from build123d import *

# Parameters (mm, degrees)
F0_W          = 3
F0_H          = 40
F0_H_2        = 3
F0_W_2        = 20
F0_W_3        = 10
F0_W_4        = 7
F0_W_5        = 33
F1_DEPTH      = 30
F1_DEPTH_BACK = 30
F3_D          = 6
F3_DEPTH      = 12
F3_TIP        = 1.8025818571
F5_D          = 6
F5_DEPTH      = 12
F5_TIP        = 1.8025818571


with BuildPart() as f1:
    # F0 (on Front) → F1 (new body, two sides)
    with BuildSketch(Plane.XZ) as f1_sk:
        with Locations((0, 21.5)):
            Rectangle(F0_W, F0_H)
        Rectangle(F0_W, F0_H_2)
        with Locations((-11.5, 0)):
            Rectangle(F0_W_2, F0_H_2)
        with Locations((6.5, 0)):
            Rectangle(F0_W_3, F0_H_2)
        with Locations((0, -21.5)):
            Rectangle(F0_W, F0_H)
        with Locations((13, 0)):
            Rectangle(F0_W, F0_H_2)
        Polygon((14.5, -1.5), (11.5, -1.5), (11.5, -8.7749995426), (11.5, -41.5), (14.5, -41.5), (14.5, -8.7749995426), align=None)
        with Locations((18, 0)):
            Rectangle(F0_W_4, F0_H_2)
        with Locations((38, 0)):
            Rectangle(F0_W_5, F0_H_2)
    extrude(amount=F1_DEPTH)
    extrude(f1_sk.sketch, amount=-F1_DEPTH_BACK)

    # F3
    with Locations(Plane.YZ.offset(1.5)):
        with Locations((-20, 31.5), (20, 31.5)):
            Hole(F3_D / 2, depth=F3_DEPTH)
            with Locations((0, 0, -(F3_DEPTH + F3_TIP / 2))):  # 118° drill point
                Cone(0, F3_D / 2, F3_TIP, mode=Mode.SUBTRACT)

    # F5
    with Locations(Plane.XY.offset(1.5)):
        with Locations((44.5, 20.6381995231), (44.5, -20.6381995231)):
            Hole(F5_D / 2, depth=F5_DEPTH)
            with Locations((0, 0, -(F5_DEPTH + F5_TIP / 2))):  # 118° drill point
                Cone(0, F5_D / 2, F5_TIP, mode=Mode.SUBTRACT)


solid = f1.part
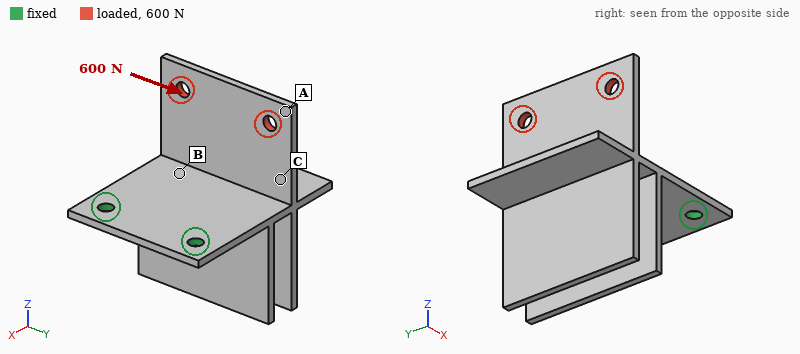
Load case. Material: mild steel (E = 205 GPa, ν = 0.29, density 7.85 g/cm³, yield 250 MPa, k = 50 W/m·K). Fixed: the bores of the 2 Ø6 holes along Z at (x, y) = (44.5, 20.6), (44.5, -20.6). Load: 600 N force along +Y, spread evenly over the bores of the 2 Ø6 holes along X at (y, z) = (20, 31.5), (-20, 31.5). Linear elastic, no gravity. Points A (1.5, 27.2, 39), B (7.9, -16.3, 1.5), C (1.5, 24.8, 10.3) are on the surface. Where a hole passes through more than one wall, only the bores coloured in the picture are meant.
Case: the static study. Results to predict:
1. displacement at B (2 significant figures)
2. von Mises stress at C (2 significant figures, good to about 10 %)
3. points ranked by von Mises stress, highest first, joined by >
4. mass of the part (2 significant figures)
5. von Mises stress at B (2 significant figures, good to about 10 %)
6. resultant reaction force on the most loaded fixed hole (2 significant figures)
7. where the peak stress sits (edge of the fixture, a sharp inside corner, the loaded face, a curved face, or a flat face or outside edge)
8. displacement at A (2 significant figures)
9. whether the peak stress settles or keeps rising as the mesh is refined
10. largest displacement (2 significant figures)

0.10 mm
34 MPa
B > C > A
270 g
80 MPa
790 N
edge of the fixture
0.36 mm
keeps rising
0.38 mm
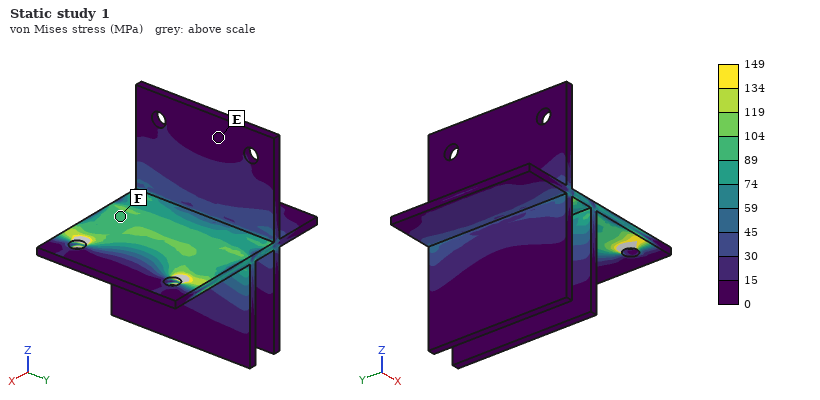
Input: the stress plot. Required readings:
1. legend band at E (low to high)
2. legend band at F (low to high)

0 to 15 MPa
89 to 104 MPa
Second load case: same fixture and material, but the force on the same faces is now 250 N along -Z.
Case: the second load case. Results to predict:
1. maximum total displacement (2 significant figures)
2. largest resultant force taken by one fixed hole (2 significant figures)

0.44 mm
130 N
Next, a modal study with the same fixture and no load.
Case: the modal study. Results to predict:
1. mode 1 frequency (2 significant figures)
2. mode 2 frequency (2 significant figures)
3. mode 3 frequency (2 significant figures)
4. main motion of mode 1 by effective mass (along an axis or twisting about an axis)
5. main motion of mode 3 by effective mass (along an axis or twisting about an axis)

280 Hz
670 Hz
990 Hz
along Z
along Z
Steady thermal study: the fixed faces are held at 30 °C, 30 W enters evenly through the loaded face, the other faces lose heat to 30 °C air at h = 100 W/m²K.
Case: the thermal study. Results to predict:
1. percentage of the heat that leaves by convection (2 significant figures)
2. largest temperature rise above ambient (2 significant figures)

97 %
78 K
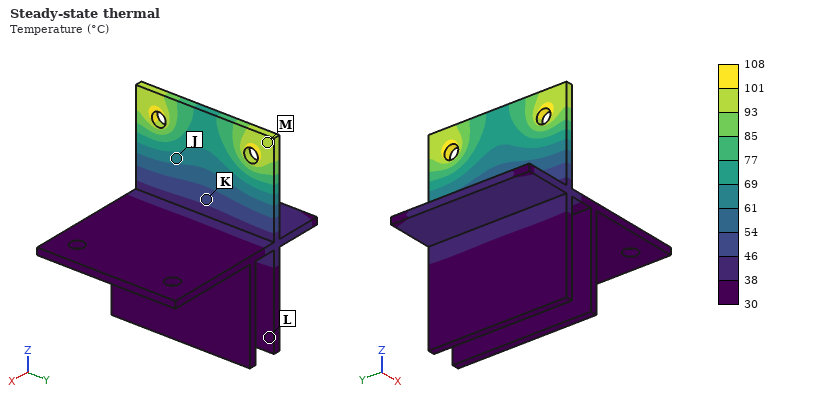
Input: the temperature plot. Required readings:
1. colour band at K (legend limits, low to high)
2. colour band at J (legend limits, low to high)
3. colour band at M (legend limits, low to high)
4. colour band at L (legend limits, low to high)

46 to 54 °C
61 to 69 °C
93 to 101 °C
30 to 38 °C
